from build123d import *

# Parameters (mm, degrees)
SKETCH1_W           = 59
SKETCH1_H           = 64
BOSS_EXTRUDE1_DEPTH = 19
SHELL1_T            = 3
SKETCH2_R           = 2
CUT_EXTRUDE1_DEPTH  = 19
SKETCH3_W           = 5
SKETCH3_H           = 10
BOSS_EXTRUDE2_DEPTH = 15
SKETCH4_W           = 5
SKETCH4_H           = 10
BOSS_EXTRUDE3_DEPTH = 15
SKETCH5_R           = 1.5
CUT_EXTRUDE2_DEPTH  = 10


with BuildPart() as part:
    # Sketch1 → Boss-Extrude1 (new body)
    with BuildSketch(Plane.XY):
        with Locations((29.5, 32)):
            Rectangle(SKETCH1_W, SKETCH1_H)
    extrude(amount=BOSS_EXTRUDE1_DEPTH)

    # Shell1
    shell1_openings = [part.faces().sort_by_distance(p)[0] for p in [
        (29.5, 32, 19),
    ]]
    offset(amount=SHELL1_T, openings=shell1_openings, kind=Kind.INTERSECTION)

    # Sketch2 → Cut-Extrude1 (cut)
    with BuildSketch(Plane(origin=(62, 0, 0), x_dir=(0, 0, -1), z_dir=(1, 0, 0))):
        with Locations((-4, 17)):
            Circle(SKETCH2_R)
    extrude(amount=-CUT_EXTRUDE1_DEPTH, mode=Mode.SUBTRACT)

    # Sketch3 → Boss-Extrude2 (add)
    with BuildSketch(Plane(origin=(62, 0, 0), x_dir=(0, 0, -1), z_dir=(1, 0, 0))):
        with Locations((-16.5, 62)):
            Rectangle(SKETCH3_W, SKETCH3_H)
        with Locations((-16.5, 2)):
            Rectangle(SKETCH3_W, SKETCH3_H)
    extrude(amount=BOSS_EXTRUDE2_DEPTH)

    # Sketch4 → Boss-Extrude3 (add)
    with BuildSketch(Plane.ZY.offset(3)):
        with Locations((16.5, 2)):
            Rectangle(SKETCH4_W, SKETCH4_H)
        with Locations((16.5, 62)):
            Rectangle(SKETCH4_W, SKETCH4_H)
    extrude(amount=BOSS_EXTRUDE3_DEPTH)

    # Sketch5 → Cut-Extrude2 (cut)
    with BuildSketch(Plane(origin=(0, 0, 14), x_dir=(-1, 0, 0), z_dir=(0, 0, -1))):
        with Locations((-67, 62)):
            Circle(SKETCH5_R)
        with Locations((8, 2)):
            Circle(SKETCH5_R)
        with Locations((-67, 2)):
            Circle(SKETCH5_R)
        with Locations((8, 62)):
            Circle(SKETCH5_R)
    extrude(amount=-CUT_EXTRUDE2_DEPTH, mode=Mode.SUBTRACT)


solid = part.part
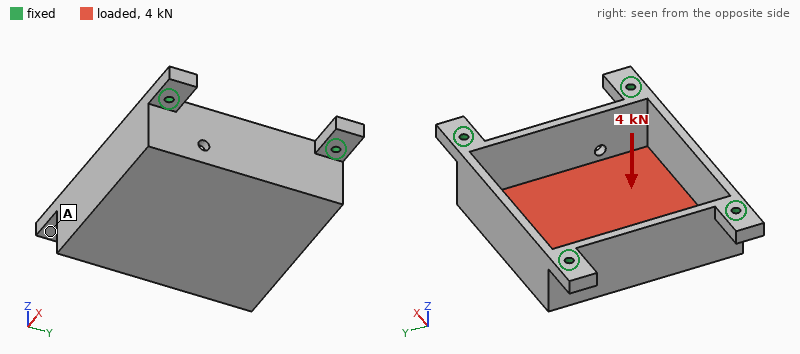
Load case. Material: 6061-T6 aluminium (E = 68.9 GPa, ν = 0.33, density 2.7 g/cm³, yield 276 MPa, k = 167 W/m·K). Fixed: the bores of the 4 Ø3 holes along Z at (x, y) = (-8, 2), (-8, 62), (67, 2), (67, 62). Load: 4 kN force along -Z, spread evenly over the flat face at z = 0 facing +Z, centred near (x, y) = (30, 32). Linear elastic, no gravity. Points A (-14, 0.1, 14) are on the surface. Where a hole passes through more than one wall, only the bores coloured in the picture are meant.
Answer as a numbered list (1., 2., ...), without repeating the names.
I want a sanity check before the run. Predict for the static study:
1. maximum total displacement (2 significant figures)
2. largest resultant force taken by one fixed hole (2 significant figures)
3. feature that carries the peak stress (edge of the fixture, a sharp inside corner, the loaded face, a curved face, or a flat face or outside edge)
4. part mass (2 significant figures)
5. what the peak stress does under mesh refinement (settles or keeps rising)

1. 0.24 mm
2. 1.2 kN
3. edge of the fixture
4. 84 g
5. keeps rising
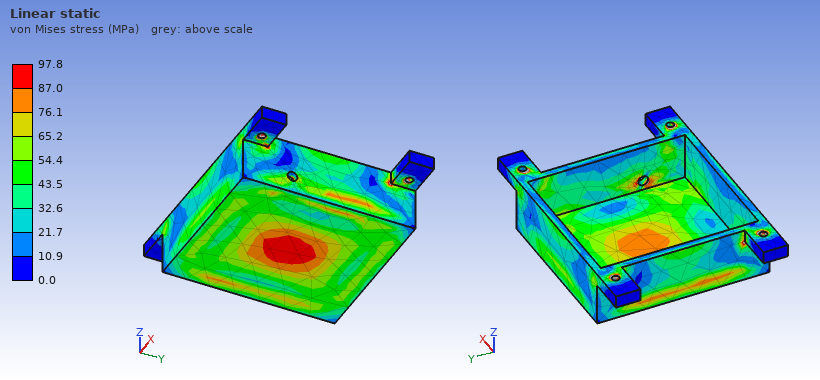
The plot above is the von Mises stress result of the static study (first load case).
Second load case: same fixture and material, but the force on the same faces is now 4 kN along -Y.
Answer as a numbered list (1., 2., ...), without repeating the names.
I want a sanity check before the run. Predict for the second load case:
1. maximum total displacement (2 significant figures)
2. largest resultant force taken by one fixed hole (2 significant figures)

1. 35 µm
2. 1.1 kN
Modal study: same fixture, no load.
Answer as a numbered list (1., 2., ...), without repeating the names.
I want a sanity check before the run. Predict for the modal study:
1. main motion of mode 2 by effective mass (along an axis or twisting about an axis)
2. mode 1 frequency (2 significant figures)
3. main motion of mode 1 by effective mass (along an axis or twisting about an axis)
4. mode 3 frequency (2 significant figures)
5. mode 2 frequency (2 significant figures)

1. along Y
2. 4400 Hz
3. along Z
4. 7200 Hz
5. 5900 Hz
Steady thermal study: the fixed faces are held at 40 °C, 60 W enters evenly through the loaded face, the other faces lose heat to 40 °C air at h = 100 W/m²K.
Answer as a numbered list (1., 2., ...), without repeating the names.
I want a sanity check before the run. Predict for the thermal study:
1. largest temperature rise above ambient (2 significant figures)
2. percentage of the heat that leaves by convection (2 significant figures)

1. 26 K
2. 42 %
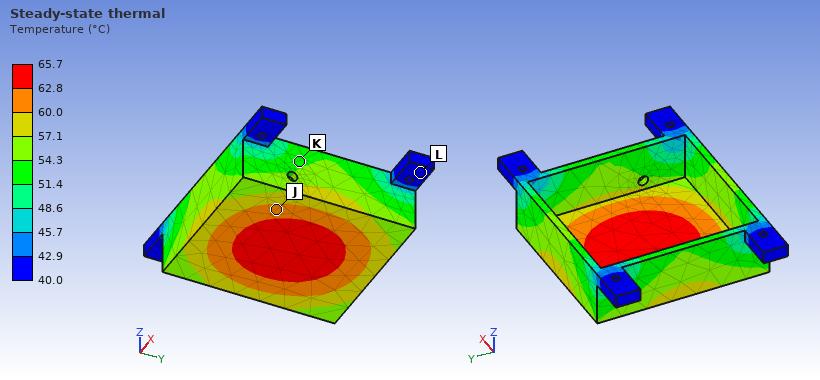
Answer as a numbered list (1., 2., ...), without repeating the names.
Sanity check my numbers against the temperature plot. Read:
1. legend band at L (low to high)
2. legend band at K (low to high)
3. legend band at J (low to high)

1. 40.0 to 42.9 °C
2. 51.4 to 54.3 °C
3. 60.0 to 62.8 °C
